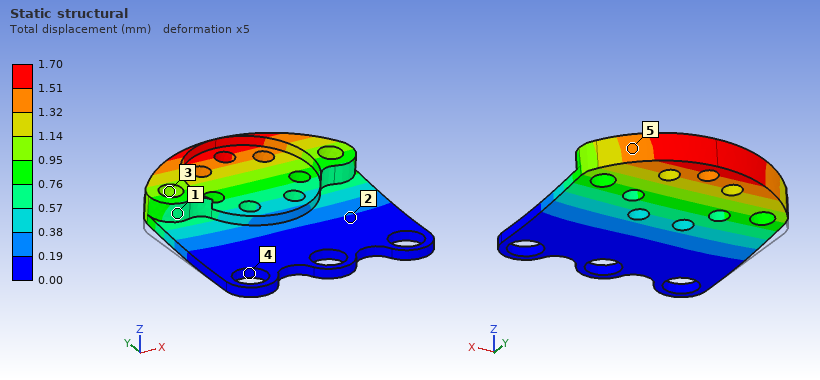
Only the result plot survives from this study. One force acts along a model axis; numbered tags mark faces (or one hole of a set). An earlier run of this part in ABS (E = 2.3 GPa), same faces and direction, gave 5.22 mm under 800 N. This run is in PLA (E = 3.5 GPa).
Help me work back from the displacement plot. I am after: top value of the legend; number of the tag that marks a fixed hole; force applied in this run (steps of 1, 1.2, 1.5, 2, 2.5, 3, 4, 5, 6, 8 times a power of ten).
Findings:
1.70 mm
4
400 N
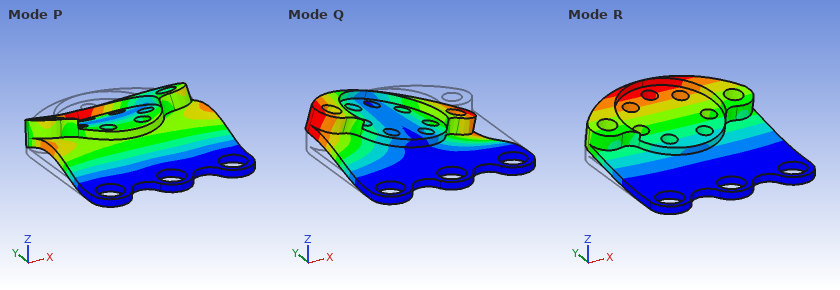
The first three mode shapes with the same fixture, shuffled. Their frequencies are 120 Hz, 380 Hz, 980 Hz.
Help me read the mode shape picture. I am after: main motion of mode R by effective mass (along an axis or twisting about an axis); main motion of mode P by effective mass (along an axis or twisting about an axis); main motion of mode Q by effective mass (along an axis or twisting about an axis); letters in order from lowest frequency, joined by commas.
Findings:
along Z
along Z
twisting about Y
R, Q, P
